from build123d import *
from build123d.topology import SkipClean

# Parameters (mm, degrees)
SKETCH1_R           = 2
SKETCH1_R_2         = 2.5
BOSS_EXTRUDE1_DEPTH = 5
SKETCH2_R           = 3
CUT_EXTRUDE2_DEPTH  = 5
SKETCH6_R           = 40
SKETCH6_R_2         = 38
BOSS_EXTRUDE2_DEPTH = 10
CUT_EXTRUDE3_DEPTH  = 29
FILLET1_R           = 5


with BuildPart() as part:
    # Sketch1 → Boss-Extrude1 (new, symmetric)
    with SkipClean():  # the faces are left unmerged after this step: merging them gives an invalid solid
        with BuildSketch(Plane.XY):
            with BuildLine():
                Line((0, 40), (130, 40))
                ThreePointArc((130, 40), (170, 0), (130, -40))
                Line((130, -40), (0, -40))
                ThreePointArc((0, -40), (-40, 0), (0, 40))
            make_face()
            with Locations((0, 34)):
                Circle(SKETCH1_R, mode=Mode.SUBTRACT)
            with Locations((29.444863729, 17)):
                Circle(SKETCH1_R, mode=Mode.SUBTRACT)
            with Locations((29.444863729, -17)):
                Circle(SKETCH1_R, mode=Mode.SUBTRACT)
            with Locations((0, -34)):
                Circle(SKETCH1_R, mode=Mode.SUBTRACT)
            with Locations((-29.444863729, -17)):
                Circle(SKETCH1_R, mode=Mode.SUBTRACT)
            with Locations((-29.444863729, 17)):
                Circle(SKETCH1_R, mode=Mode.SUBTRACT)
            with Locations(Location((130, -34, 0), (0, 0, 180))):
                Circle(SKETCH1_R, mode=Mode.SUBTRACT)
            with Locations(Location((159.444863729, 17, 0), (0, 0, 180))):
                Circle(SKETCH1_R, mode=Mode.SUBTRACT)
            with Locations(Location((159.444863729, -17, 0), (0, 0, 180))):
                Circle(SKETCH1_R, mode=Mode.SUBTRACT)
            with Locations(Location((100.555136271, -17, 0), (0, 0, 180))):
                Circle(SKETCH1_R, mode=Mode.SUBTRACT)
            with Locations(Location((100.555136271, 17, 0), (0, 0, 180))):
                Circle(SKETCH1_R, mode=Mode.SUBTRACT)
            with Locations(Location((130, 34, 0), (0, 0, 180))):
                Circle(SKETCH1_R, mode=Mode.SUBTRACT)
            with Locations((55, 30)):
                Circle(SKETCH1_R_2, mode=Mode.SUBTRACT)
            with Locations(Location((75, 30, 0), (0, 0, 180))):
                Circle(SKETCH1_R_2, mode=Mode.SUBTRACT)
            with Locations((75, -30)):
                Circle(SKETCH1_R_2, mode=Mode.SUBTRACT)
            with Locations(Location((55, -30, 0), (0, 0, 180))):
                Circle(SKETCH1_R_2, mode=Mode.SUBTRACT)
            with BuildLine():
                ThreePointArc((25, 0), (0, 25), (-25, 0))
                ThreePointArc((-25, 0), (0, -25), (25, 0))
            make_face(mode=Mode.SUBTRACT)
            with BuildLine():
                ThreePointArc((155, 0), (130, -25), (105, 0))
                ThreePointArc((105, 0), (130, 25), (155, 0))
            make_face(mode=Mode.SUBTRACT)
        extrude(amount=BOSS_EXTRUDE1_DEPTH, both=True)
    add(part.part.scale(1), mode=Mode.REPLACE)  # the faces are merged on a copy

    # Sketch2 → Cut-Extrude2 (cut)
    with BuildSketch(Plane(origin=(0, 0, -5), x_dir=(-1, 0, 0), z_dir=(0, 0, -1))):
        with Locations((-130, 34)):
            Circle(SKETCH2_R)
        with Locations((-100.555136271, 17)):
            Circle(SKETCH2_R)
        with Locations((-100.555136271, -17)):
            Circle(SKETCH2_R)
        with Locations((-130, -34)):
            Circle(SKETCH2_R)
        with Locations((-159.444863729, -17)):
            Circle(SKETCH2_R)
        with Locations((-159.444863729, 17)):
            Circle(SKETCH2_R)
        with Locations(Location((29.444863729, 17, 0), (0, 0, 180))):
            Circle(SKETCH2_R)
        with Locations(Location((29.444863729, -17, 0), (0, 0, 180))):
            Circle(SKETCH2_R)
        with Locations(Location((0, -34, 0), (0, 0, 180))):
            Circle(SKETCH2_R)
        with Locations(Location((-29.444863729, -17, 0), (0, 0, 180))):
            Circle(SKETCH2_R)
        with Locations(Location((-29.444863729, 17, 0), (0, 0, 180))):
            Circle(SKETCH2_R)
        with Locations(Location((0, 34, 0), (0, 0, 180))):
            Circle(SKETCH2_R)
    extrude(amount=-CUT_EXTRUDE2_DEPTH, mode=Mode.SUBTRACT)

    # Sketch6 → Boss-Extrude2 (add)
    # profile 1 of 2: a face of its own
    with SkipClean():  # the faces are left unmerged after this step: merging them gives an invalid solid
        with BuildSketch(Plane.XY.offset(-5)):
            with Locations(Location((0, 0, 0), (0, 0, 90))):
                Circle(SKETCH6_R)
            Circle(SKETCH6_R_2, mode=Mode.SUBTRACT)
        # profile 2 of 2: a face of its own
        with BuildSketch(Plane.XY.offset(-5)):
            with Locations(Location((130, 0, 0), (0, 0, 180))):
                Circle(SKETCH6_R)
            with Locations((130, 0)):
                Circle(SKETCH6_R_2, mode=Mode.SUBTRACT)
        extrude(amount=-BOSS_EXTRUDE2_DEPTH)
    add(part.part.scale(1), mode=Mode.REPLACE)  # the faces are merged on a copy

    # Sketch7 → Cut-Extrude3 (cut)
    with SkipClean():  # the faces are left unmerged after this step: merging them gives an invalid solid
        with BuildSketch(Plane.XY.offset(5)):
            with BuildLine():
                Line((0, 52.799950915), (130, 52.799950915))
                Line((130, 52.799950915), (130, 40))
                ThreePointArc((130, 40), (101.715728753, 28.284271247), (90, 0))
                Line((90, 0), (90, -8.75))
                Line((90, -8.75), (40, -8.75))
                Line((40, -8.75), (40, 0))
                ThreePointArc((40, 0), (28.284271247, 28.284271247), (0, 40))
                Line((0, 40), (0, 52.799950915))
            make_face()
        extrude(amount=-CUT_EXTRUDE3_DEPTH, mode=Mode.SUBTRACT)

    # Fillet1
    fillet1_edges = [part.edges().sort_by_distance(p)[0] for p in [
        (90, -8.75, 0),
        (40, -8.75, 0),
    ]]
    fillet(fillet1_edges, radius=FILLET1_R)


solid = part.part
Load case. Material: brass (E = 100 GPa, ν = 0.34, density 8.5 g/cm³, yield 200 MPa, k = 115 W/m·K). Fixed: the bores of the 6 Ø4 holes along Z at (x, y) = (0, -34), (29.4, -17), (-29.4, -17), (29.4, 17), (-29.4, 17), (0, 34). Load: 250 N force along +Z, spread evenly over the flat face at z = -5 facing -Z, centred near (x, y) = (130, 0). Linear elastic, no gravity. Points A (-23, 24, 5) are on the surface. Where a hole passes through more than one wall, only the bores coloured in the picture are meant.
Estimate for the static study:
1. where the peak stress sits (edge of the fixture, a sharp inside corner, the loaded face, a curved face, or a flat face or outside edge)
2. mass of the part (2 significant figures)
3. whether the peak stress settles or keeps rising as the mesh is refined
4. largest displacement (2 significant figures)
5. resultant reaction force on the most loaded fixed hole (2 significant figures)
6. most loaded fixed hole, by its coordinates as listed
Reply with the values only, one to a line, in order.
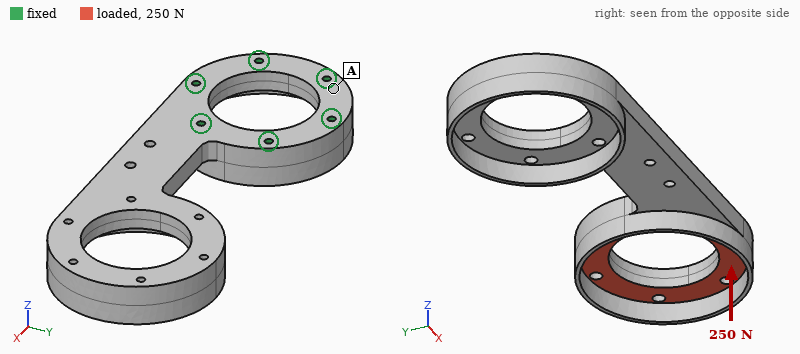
edge of the fixture
770 g
keeps rising
0.66 mm
1.1 kN
(29.4, -17)
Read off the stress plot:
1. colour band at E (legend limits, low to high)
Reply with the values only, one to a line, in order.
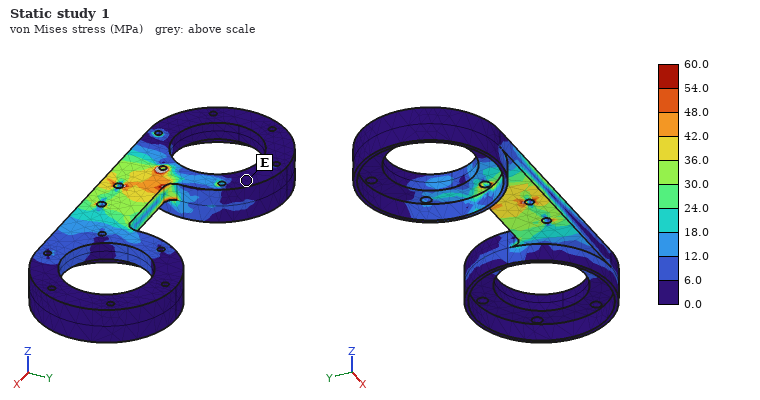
0.0 to 6.0 MPa
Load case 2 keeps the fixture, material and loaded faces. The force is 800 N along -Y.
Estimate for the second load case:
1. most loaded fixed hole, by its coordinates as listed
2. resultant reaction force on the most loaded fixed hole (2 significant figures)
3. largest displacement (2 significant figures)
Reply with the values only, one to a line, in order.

(0, -34)
1.8 kN
0.26 mm
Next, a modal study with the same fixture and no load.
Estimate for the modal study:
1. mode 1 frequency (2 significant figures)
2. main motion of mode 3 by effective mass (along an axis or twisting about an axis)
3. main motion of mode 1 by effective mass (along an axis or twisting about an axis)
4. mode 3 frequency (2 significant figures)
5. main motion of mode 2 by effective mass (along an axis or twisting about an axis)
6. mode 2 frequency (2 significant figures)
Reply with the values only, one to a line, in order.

210 Hz
twisting about X
along Z
650 Hz
along Y
570 Hz
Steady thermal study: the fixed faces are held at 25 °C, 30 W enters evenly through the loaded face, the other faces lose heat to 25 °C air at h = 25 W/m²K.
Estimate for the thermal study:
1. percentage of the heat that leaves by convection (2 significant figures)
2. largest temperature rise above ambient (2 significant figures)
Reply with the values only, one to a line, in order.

55 %
49 K
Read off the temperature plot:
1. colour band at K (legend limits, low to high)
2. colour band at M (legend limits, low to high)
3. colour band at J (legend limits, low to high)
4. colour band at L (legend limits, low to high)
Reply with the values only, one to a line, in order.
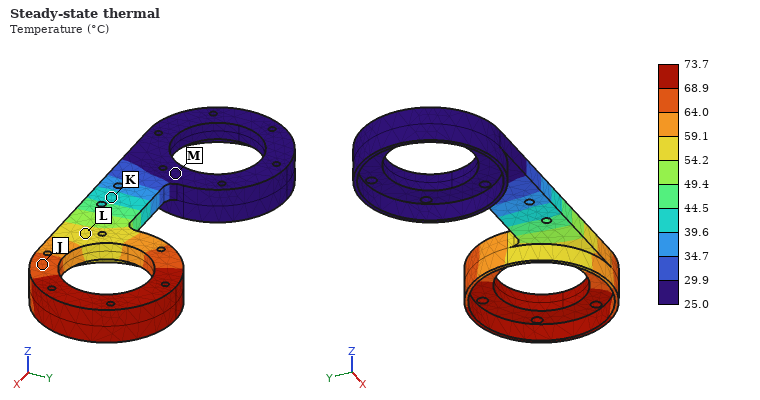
39.6 to 44.5 °C
25.0 to 29.9 °C
64.0 to 68.9 °C
54.2 to 59.1 °C
